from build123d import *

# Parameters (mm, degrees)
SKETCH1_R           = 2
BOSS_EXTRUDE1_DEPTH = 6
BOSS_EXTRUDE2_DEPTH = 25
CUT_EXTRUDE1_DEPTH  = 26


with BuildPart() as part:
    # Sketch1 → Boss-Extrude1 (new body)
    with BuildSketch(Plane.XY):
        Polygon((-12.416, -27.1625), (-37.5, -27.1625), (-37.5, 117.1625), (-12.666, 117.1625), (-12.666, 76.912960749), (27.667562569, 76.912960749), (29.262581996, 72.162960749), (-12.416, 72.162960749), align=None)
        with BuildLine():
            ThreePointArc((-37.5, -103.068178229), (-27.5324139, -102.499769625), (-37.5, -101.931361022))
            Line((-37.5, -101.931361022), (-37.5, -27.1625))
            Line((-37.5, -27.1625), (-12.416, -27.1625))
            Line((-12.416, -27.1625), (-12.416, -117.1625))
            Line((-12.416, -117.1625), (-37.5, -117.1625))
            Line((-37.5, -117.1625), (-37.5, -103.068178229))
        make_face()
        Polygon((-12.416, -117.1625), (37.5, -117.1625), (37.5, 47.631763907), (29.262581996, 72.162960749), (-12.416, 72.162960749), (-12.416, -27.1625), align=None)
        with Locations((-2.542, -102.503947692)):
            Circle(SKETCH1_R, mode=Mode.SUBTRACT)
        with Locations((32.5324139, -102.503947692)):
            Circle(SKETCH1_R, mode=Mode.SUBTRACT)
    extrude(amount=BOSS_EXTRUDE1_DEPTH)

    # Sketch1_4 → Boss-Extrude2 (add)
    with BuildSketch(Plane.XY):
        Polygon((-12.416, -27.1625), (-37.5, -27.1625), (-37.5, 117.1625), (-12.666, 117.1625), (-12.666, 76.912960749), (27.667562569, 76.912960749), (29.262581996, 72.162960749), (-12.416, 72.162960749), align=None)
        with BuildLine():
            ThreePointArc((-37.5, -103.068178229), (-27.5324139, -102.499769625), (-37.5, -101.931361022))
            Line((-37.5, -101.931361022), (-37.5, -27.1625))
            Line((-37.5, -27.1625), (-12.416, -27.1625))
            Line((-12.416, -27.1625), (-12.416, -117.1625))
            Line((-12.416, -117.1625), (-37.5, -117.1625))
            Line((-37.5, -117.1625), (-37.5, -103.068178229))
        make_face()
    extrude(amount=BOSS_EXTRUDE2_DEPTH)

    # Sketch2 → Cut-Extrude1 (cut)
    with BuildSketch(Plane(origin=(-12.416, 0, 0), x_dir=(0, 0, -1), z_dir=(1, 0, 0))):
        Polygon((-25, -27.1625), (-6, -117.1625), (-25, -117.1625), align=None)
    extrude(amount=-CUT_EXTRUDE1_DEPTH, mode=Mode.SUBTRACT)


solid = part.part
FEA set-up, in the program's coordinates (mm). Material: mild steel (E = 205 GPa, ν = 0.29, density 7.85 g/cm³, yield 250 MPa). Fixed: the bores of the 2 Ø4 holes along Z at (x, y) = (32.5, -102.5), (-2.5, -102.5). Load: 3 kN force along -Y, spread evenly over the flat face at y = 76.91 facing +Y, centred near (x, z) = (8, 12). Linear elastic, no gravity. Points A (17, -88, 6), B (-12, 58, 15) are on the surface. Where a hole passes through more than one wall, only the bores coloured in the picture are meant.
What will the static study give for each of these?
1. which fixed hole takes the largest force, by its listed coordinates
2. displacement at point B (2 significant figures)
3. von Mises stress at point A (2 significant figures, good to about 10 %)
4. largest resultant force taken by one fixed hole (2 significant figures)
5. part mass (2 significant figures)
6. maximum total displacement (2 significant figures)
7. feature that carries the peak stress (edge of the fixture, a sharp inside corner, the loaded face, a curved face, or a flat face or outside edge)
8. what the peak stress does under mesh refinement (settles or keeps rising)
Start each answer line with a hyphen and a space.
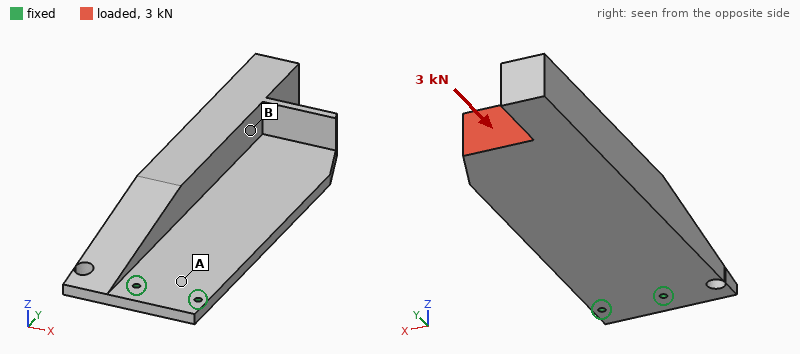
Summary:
- (-2.5, -102.5)
- 0.41 mm
- 41 MPa
- 2.1 kN
- 1.5 kg
- 0.60 mm
- edge of the fixture
- keeps rising
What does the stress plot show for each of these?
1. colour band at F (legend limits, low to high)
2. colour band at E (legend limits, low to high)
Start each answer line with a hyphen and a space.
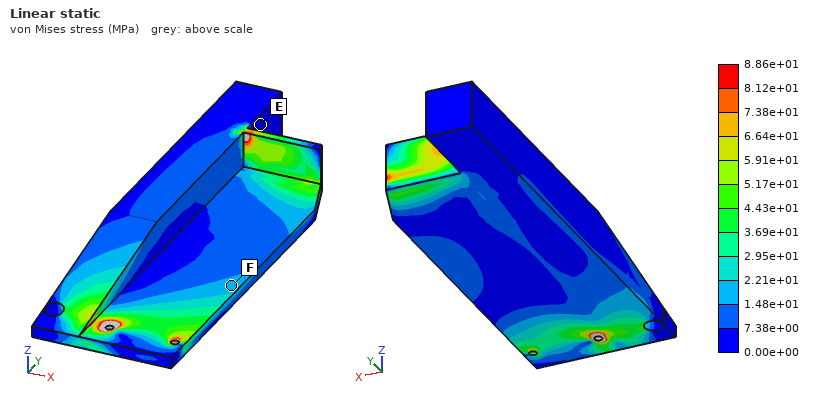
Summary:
- 1.48e+01 to 2.21e+01 MPa
- 0.00e+00 to 7.38e+00 MPa
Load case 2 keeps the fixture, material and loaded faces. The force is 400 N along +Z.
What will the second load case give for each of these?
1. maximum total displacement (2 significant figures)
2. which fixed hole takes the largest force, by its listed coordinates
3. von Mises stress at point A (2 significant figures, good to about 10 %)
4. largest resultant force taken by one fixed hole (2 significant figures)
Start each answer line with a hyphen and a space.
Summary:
- 1.4 mm
- (-2.5, -102.5)
- 91 MPa
- 320 N
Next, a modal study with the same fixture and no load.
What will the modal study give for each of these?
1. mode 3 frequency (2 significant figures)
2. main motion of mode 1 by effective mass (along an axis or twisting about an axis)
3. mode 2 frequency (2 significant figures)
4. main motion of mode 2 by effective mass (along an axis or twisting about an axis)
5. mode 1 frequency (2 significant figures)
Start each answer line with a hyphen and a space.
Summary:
- 820 Hz
- along Z
- 610 Hz
- along X
- 110 Hz
